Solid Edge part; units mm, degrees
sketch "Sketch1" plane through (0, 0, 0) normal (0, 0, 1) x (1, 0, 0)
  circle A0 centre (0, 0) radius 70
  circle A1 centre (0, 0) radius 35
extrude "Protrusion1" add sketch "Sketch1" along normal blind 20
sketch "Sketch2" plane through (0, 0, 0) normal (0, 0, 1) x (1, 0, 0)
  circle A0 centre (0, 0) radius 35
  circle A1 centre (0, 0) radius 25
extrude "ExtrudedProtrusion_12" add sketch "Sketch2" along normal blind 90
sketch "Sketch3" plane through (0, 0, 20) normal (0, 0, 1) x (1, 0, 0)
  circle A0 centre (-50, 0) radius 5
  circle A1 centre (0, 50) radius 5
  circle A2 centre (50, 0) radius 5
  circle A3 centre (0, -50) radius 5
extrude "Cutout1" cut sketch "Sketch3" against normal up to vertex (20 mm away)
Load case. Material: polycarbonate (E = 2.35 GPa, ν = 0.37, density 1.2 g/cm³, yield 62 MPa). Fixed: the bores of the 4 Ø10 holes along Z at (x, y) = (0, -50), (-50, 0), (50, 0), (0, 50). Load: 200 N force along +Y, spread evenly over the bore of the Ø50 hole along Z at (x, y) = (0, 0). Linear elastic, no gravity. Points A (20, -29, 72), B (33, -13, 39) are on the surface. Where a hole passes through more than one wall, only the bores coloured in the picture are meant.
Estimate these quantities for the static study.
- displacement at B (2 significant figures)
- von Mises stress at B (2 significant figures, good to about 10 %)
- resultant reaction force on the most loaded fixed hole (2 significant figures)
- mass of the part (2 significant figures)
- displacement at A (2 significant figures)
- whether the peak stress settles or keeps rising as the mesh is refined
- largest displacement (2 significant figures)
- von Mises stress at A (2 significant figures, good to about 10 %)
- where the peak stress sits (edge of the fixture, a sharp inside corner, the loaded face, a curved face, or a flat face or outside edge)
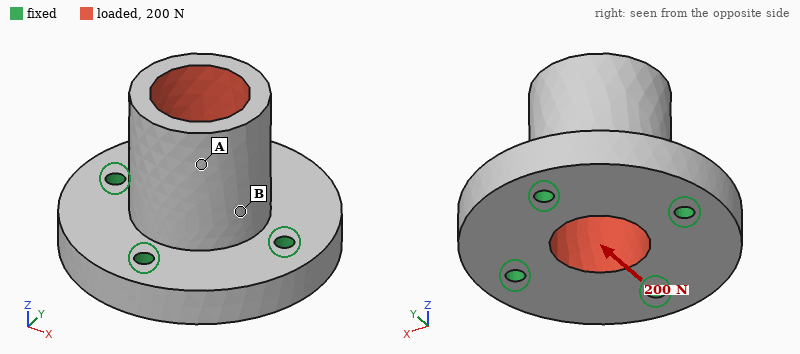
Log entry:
6.2 µm
0.14 MPa
93 N
470 g
14 µm
keeps rising
18 µm
0.053 MPa
edge of the fixture
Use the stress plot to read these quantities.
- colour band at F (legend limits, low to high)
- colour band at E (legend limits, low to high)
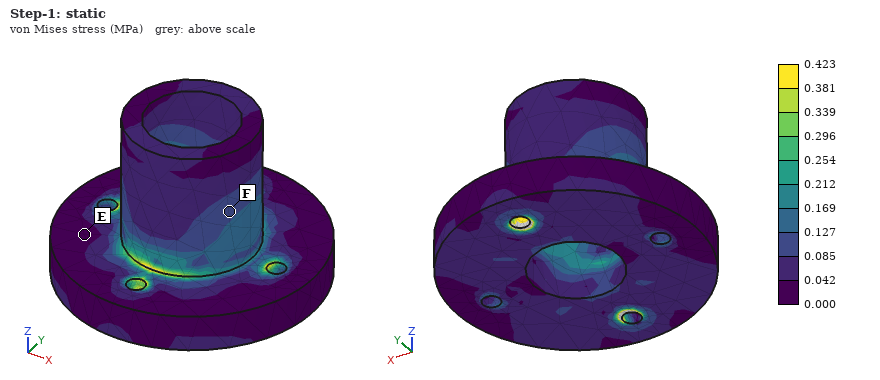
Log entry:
0.085 to 0.127 MPa
0.000 to 0.042 MPa
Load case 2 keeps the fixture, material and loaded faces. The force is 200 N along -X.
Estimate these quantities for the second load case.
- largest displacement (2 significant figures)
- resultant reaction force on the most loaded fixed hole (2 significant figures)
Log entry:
18 µm
94 N
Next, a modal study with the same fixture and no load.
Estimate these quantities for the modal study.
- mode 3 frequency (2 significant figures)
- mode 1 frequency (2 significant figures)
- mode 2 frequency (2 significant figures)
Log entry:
2100 Hz
1400 Hz
1400 Hz
